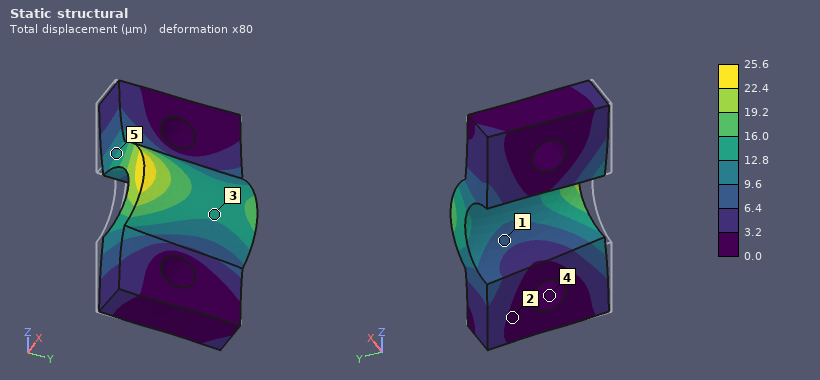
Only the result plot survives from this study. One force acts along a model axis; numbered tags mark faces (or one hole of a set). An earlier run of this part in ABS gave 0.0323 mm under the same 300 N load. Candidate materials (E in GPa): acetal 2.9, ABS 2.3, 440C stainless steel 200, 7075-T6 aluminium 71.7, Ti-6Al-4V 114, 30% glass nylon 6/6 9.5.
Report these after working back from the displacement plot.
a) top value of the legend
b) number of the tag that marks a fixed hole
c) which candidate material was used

25.6 µm
4
acetal
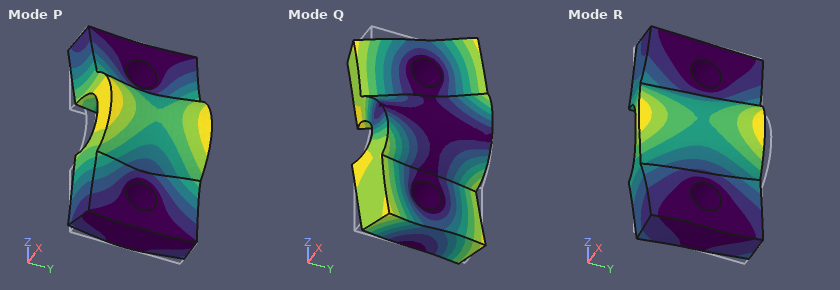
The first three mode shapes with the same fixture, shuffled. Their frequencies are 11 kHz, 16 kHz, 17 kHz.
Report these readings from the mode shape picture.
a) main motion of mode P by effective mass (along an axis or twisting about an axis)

along X
